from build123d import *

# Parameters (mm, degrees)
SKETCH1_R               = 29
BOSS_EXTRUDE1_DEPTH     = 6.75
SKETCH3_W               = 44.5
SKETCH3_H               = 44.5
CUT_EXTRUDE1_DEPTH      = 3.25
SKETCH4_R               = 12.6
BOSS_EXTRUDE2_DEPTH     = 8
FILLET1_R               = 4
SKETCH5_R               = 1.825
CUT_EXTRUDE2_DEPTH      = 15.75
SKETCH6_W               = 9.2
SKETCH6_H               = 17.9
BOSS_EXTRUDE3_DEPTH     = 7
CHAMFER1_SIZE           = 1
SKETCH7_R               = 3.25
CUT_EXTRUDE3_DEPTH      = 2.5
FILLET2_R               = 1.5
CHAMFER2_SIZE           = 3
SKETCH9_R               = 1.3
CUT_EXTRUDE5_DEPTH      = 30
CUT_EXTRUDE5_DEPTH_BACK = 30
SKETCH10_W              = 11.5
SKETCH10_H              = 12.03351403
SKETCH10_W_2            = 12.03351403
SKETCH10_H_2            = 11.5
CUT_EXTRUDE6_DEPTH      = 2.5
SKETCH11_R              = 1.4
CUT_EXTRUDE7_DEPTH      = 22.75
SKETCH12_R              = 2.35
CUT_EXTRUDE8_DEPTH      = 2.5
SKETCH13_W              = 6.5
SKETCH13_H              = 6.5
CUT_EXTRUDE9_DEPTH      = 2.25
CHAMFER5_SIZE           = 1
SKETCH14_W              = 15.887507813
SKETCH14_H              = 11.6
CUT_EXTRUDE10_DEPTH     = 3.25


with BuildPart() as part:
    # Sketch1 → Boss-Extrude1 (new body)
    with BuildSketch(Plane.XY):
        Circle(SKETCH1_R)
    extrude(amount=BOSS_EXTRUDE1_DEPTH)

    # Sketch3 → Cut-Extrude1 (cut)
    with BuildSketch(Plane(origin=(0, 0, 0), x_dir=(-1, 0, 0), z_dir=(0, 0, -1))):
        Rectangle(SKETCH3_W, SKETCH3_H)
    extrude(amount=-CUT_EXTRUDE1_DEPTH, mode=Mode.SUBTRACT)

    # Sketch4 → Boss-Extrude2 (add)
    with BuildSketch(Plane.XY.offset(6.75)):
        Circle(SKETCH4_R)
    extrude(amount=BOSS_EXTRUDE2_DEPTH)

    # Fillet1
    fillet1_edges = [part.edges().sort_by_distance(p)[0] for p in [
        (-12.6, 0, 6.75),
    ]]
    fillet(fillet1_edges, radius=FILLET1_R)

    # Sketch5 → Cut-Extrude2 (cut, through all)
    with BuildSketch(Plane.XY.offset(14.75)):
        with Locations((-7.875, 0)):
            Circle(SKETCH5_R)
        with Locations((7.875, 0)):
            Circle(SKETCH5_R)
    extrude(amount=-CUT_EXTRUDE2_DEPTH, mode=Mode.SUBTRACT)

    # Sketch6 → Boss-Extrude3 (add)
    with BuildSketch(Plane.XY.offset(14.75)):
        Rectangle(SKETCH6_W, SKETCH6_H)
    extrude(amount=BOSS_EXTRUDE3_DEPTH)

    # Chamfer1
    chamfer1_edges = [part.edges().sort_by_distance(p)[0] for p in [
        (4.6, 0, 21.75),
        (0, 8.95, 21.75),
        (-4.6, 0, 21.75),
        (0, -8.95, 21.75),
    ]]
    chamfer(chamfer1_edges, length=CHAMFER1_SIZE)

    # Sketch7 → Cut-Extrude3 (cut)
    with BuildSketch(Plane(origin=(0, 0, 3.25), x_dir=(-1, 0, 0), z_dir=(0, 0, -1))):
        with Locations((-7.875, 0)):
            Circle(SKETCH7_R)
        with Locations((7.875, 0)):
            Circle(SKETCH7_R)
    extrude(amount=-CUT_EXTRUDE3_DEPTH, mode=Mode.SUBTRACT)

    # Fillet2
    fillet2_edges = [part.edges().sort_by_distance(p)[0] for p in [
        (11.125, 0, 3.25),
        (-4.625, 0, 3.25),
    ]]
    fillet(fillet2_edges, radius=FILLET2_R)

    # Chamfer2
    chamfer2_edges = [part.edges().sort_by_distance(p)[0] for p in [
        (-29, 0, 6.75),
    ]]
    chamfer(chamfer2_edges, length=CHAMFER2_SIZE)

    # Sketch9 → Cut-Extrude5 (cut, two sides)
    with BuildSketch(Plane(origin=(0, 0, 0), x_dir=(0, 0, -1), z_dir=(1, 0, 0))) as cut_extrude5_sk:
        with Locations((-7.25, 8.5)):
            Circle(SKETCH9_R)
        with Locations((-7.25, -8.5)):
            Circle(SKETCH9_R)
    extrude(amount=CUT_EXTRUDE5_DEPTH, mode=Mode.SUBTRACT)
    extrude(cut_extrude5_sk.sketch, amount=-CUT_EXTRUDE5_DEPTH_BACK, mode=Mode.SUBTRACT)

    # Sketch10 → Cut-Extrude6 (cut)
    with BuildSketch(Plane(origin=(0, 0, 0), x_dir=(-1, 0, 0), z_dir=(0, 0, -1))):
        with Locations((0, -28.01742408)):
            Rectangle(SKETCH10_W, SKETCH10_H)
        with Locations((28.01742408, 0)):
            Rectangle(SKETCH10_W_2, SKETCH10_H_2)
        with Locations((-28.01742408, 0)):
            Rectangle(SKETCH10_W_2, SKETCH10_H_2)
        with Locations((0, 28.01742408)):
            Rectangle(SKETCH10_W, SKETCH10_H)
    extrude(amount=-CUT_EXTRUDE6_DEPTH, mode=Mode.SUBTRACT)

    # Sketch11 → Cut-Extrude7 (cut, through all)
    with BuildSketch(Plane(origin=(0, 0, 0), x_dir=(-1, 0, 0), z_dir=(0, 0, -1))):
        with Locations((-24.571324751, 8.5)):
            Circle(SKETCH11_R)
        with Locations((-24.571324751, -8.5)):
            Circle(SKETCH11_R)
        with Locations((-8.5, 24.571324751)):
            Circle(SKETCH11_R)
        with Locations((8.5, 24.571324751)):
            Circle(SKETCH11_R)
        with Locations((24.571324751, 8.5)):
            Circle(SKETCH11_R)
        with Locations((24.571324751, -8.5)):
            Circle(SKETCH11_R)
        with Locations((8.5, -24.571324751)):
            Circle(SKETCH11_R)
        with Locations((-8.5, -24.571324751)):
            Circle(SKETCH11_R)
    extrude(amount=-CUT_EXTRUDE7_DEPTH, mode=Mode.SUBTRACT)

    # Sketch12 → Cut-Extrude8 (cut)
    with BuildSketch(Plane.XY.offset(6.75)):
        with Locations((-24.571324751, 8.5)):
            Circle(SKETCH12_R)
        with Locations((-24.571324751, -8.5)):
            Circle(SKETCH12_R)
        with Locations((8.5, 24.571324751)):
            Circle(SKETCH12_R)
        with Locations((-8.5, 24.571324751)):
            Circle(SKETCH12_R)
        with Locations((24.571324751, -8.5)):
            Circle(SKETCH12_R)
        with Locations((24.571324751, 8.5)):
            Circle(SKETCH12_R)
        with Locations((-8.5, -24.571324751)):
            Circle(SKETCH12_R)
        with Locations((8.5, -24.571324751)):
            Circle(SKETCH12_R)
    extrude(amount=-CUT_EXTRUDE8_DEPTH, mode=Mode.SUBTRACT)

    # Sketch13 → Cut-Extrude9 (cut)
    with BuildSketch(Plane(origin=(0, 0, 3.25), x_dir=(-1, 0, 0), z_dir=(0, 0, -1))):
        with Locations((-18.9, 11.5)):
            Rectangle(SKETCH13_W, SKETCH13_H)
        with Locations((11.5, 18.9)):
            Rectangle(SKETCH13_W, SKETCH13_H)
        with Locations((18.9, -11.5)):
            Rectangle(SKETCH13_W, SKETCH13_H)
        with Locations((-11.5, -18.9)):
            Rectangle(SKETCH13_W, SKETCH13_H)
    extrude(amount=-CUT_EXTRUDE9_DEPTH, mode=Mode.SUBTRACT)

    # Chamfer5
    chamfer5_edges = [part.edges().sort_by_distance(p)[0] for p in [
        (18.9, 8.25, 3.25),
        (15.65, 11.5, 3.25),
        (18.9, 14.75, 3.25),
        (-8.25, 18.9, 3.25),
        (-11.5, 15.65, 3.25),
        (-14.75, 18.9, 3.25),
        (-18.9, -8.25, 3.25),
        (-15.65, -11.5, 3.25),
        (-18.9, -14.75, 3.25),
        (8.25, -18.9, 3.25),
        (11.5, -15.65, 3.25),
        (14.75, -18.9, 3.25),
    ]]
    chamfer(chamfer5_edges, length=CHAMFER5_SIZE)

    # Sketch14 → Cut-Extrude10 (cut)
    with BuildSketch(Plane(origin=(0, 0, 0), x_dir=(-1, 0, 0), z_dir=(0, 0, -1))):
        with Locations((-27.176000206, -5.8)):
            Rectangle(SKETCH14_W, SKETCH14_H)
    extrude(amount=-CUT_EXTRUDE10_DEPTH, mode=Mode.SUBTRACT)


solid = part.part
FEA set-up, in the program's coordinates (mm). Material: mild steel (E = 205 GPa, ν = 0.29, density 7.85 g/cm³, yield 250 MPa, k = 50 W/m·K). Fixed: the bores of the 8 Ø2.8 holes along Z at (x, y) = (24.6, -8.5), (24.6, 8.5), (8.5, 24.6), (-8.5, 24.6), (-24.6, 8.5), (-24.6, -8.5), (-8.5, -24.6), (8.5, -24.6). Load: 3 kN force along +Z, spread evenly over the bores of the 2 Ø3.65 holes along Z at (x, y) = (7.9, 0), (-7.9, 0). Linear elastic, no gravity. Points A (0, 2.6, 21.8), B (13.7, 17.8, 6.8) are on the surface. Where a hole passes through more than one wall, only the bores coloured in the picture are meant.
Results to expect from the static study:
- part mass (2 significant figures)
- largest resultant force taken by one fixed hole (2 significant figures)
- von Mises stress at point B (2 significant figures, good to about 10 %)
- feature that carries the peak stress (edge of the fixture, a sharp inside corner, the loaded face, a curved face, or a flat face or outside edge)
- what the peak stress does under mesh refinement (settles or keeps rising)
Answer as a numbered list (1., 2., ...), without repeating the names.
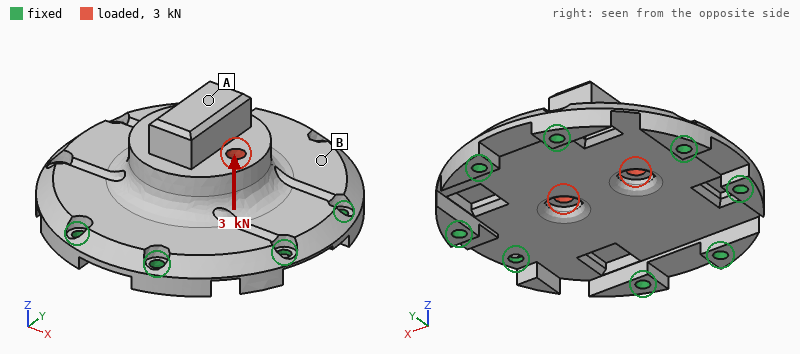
1. 110 g
2. 860 N
3. 28 MPa
4. edge of the fixture
5. keeps rising
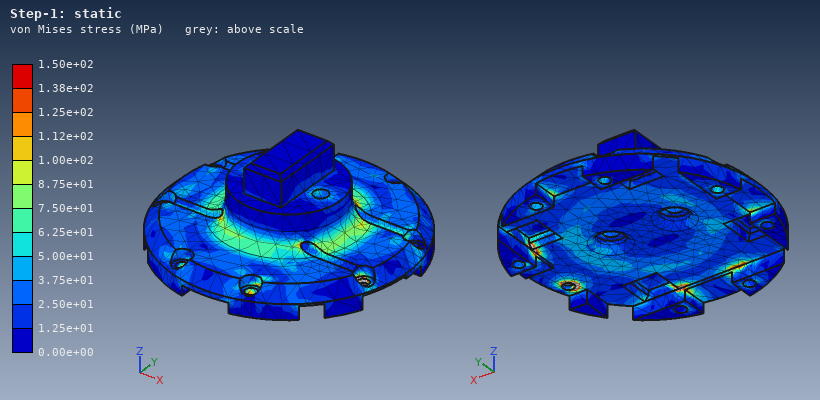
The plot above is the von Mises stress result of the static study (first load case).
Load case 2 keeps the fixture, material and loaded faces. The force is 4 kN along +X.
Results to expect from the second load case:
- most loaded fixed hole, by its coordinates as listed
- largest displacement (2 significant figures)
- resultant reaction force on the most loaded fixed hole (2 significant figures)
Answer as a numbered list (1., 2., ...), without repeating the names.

1. (-24.6, 8.5)
2. 6.7 µm
3. 940 N
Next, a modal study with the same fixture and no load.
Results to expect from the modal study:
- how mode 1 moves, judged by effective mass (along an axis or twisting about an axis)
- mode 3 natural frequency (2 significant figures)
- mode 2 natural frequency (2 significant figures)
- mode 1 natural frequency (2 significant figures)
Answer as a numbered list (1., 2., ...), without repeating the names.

1. along Z
2. 15 kHz
3. 15 kHz
4. 9800 Hz
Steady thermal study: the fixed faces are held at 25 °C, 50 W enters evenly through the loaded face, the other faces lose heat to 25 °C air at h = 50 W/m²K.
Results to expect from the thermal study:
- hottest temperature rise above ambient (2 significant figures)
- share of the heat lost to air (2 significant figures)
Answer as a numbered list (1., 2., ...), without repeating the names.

1. 66 K
2. 20 %
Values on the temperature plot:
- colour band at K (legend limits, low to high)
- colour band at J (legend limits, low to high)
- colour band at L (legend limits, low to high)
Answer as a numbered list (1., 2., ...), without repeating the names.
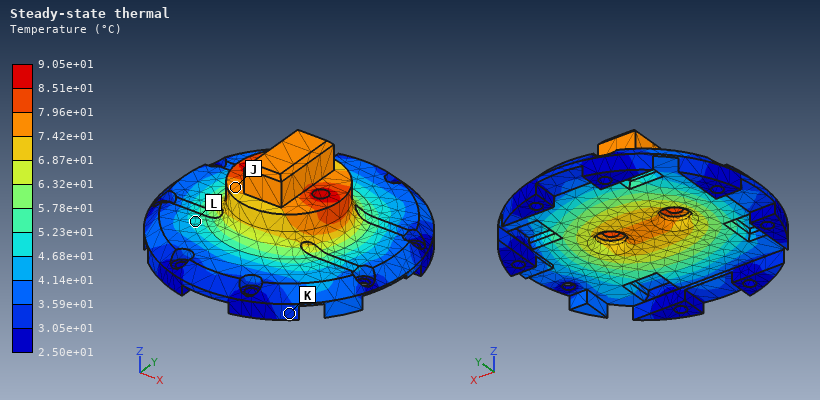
1. 3.05e+01 to 3.59e+01 °C
2. 7.42e+01 to 7.96e+01 °C
3. 4.68e+01 to 5.23e+01 °C
